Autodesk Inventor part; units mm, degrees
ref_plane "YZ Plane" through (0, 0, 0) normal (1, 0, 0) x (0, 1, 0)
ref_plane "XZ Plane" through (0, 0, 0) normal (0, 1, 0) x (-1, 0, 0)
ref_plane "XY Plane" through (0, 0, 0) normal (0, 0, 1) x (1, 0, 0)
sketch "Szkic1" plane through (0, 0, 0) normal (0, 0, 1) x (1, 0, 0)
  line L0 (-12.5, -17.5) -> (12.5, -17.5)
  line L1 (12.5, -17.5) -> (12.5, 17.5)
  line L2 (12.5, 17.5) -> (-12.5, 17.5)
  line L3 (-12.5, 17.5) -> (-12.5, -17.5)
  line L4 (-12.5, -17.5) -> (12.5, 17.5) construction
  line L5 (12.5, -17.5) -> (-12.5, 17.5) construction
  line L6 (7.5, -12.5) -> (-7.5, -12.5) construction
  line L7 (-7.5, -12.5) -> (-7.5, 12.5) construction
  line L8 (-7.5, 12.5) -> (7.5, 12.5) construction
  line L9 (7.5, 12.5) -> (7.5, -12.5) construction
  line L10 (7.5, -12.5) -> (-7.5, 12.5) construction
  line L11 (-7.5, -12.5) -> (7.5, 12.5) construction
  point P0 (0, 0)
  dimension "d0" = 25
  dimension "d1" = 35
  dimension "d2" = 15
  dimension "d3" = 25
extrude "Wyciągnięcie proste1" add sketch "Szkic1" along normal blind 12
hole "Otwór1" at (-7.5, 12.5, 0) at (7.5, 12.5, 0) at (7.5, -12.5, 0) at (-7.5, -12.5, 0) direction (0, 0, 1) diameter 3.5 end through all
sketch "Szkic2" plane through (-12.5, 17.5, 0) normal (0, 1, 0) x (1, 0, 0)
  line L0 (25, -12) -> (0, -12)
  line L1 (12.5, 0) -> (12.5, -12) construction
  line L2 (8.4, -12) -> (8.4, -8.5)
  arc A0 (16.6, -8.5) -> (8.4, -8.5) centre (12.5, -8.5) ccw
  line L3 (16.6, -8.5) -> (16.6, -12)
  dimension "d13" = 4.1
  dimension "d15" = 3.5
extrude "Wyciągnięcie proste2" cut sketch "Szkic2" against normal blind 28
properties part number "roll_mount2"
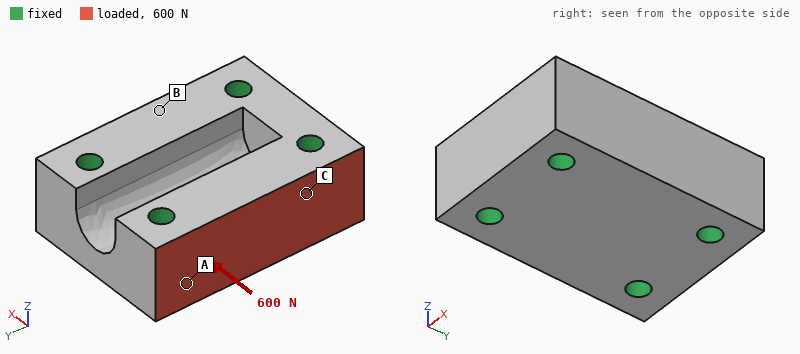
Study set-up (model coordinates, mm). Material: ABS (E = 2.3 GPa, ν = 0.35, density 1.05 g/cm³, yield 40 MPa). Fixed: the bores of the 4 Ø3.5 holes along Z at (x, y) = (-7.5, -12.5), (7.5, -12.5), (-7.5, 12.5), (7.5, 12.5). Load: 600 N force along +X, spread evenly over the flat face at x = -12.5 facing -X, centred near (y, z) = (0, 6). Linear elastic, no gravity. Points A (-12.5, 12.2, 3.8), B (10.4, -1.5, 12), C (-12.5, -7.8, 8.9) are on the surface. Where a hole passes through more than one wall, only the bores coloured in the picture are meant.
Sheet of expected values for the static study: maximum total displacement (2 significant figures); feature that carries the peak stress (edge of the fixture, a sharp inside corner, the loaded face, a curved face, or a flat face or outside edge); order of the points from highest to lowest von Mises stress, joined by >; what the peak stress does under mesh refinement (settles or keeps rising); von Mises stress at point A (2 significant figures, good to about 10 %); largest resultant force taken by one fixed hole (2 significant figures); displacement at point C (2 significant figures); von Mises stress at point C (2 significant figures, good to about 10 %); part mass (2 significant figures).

25 µm
edge of the fixture
A > C > B
keeps rising
2.9 MPa
250 N
12 µm
1.7 MPa
8.9 g
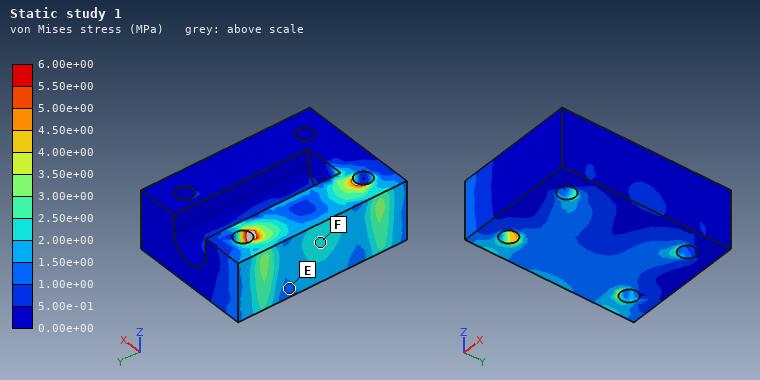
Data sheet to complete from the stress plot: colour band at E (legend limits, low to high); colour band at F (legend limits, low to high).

1.00e+00 to 1.50e+00 MPa
2.00e+00 to 2.50e+00 MPa
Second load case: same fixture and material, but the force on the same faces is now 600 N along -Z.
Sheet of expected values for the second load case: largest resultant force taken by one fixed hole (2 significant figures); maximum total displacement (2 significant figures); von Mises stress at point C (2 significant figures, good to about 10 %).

310 N
51 µm
5.7 MPa
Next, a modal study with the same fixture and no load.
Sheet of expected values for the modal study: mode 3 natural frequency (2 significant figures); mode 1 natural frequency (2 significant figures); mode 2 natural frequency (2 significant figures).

16 kHz
15 kHz
15 kHz
